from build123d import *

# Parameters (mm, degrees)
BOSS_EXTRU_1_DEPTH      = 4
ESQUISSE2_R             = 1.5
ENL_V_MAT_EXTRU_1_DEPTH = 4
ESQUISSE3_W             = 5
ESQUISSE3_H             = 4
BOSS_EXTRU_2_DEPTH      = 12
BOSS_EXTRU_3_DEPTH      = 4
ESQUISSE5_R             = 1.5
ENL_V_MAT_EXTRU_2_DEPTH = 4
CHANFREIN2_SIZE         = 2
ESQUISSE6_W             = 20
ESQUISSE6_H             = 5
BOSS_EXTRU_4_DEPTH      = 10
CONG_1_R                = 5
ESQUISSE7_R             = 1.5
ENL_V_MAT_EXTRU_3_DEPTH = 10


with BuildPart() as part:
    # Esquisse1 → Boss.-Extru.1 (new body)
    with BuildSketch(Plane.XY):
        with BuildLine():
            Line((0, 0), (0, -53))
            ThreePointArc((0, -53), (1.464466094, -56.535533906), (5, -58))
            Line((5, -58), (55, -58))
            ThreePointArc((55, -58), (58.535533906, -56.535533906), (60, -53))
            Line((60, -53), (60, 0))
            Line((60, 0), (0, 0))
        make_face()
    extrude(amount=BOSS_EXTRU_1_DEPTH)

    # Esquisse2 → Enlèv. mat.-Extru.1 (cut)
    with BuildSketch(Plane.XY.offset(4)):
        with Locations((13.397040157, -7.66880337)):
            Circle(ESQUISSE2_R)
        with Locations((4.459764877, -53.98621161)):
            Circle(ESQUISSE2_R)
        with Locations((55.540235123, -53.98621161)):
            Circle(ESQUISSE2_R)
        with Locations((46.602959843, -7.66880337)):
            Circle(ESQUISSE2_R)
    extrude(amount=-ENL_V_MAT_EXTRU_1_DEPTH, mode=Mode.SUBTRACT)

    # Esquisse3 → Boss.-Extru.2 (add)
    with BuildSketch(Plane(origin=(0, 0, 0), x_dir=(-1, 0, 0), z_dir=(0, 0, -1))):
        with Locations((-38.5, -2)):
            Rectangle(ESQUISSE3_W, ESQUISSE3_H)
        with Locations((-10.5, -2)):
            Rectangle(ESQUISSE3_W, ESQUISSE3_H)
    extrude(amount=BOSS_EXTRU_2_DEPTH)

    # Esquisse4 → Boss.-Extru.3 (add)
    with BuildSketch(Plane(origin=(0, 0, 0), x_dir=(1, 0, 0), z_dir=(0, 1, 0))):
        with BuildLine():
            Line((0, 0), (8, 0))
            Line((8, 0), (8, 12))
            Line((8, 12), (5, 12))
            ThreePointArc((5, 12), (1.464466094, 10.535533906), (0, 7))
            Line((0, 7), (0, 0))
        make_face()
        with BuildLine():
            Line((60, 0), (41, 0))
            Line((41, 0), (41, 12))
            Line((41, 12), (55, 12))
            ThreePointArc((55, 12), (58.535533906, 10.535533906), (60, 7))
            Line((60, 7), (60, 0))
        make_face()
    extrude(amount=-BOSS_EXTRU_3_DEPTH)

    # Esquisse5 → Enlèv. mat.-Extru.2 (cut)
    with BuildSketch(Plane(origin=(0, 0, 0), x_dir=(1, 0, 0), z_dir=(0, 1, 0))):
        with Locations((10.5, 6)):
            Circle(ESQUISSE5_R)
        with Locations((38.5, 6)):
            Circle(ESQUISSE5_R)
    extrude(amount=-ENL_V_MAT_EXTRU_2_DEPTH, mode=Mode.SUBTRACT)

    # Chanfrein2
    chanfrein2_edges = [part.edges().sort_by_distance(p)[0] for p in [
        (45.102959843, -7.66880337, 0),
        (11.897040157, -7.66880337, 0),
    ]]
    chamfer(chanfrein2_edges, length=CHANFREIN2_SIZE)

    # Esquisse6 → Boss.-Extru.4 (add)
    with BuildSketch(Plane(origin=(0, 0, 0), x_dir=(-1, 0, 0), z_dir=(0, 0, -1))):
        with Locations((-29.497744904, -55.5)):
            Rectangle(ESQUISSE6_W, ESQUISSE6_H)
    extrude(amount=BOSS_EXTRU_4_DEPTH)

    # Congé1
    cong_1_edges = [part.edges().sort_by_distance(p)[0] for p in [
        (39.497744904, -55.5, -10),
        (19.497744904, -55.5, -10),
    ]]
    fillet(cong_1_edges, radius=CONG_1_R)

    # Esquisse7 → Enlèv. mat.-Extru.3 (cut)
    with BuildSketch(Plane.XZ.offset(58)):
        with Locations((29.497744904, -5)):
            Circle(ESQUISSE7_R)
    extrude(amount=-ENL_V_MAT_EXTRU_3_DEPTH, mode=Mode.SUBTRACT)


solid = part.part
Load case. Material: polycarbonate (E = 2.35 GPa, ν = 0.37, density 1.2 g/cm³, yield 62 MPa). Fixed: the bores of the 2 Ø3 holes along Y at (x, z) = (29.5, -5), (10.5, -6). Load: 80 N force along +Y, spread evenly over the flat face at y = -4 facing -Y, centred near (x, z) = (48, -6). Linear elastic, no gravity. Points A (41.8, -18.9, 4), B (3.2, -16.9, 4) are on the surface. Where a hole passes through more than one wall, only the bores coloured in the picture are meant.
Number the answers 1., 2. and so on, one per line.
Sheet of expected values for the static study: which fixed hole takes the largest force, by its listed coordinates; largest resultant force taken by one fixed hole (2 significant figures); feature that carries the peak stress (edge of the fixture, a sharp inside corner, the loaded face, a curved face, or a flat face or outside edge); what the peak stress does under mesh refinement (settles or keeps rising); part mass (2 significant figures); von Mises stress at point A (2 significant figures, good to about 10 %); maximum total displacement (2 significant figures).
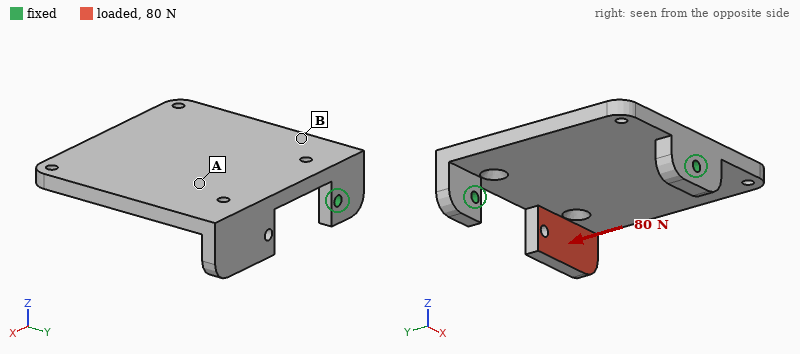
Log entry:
1. (29.5, -5)
2. 73 N
3. edge of the fixture
4. keeps rising
5. 20 g
6. 3.1 MPa
7. 0.97 mm
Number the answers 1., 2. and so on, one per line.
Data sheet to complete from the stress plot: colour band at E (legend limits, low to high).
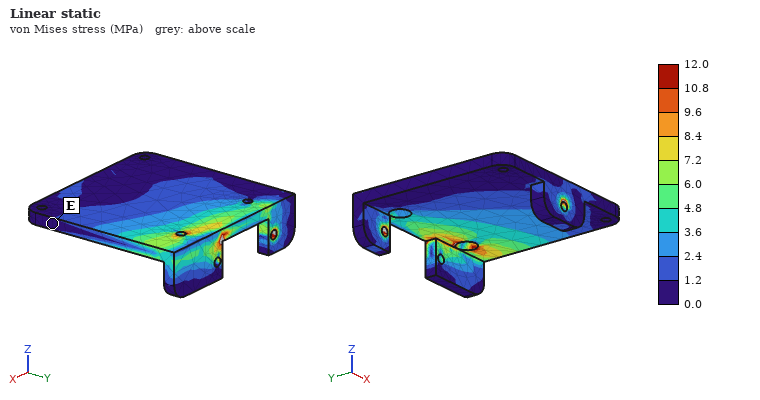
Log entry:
1. 0.0 to 1.2 MPa
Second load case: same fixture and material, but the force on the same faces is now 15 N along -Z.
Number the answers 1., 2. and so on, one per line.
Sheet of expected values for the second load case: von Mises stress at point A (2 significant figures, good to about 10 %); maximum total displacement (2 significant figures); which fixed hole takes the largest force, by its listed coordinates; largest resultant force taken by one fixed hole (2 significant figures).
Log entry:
1. 2.0 MPa
2. 0.95 mm
3. (10.5, -6)
4. 14 N
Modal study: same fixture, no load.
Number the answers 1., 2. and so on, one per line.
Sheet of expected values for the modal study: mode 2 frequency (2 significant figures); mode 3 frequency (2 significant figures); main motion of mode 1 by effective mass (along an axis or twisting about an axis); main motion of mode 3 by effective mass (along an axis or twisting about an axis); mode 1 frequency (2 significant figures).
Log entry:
1. 1000 Hz
2. 1200 Hz
3. along Z
4. along Z
5. 350 Hz
